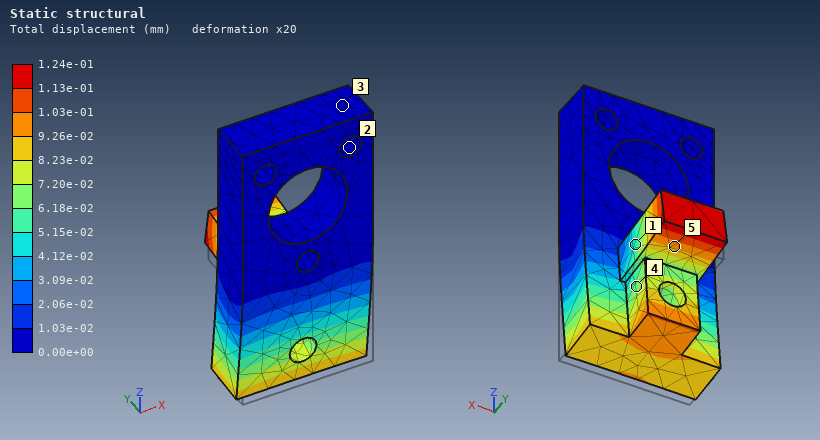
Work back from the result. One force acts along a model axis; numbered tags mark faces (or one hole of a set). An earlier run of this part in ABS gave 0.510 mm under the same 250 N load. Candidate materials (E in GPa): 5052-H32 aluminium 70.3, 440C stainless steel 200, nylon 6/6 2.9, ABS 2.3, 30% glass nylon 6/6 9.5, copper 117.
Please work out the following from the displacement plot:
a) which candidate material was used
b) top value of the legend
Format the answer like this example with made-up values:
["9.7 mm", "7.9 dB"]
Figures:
["30% glass nylon 6/6", "1.24e-01 mm"]
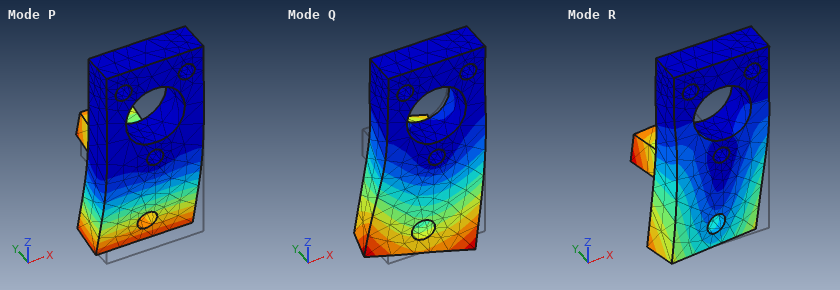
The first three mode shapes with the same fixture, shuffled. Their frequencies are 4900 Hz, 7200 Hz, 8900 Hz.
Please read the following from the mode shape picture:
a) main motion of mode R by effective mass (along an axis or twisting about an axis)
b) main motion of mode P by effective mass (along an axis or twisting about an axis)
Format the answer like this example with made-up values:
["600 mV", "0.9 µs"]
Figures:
["along X", "along Y"]
